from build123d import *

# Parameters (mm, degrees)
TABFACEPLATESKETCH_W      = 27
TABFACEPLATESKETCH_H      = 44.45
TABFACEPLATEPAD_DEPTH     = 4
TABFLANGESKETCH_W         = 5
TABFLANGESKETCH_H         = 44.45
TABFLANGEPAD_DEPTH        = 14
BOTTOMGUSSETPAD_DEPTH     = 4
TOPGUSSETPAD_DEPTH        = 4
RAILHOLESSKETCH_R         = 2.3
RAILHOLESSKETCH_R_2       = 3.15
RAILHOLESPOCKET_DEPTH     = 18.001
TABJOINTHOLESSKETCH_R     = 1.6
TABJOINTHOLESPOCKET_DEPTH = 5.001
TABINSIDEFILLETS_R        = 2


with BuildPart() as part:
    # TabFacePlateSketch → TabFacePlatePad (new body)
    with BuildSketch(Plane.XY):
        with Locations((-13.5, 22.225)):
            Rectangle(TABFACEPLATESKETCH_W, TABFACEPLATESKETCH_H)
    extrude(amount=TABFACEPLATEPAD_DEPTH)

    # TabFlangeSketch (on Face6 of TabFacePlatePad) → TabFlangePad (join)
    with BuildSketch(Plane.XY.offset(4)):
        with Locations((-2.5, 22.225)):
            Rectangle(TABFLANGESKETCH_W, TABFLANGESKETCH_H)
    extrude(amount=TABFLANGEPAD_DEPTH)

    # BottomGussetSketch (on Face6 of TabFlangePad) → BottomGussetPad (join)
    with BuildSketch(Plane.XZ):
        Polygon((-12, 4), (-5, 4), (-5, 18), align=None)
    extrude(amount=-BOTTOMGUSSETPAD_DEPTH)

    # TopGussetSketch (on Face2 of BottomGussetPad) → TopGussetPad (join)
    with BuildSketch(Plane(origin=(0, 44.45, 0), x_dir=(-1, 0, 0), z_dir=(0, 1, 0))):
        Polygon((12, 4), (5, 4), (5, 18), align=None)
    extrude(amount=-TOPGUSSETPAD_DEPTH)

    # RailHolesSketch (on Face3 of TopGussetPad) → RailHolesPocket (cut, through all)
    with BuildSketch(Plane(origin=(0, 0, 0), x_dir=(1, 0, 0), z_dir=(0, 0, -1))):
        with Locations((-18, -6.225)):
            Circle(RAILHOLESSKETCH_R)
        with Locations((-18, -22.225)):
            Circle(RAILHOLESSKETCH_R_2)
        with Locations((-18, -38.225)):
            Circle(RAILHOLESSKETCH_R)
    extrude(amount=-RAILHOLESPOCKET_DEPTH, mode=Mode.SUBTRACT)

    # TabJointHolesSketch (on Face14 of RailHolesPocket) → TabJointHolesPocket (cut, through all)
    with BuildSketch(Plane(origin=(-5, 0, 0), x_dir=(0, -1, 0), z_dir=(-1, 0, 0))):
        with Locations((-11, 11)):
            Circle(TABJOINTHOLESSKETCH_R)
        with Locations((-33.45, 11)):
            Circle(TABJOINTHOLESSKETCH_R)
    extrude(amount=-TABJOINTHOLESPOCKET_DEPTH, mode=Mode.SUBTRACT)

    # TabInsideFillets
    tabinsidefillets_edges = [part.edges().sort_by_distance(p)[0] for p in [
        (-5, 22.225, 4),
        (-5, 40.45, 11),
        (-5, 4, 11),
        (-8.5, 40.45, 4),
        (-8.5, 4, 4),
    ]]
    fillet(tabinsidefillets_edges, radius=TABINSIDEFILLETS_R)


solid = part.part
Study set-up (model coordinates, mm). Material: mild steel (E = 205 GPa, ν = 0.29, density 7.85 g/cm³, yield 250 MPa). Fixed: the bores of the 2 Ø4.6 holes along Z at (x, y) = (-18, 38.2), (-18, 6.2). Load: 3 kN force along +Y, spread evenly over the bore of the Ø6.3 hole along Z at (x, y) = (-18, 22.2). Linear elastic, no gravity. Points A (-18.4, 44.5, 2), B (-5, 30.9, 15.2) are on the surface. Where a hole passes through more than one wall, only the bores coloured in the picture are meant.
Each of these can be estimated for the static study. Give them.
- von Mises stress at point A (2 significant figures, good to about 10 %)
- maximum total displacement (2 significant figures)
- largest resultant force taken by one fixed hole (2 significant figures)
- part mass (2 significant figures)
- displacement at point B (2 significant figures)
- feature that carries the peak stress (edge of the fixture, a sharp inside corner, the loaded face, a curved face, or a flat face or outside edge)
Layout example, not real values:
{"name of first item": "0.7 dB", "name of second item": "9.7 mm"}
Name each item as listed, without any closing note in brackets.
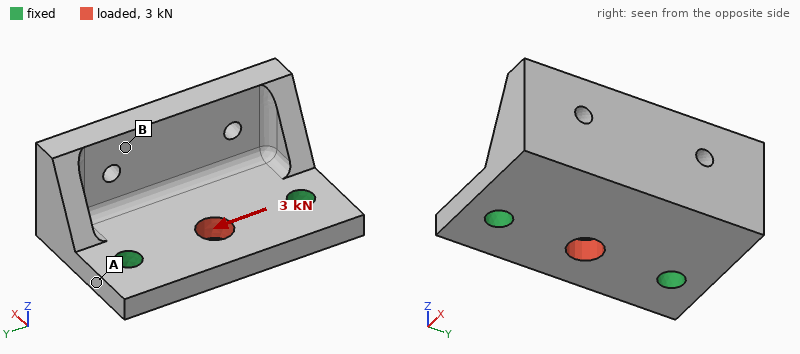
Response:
{"von Mises stress at point A": "17 MPa", "maximum total displacement": "2.3 µm", "largest resultant force taken by one fixed hole": "1.5 kN", "part mass": "63 g", "displacement at point B": "0.93 µm", "feature that carries the peak stress": "the loaded face"}
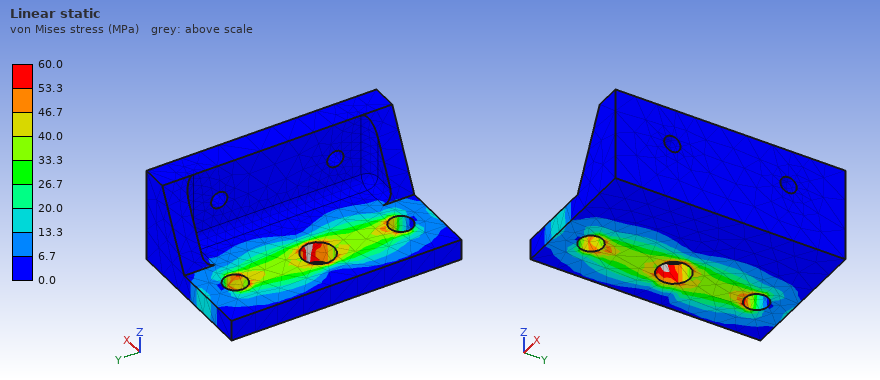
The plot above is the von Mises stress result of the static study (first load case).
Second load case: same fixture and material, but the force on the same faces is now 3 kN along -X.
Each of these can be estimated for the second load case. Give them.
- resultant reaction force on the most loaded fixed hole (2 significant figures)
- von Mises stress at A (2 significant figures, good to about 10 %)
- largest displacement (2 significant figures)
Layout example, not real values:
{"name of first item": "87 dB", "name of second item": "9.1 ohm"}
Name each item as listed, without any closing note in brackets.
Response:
{"resultant reaction force on the most loaded fixed hole": "1.5 kN", "von Mises stress at A": "15 MPa", "largest displacement": "5.2 µm"}
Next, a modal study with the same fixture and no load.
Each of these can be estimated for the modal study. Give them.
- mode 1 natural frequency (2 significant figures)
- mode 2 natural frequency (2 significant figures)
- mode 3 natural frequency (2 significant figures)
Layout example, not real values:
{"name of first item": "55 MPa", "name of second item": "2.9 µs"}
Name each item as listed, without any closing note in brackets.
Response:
{"mode 1 natural frequency": "4100 Hz", "mode 2 natural frequency": "7900 Hz", "mode 3 natural frequency": "16 kHz"}
